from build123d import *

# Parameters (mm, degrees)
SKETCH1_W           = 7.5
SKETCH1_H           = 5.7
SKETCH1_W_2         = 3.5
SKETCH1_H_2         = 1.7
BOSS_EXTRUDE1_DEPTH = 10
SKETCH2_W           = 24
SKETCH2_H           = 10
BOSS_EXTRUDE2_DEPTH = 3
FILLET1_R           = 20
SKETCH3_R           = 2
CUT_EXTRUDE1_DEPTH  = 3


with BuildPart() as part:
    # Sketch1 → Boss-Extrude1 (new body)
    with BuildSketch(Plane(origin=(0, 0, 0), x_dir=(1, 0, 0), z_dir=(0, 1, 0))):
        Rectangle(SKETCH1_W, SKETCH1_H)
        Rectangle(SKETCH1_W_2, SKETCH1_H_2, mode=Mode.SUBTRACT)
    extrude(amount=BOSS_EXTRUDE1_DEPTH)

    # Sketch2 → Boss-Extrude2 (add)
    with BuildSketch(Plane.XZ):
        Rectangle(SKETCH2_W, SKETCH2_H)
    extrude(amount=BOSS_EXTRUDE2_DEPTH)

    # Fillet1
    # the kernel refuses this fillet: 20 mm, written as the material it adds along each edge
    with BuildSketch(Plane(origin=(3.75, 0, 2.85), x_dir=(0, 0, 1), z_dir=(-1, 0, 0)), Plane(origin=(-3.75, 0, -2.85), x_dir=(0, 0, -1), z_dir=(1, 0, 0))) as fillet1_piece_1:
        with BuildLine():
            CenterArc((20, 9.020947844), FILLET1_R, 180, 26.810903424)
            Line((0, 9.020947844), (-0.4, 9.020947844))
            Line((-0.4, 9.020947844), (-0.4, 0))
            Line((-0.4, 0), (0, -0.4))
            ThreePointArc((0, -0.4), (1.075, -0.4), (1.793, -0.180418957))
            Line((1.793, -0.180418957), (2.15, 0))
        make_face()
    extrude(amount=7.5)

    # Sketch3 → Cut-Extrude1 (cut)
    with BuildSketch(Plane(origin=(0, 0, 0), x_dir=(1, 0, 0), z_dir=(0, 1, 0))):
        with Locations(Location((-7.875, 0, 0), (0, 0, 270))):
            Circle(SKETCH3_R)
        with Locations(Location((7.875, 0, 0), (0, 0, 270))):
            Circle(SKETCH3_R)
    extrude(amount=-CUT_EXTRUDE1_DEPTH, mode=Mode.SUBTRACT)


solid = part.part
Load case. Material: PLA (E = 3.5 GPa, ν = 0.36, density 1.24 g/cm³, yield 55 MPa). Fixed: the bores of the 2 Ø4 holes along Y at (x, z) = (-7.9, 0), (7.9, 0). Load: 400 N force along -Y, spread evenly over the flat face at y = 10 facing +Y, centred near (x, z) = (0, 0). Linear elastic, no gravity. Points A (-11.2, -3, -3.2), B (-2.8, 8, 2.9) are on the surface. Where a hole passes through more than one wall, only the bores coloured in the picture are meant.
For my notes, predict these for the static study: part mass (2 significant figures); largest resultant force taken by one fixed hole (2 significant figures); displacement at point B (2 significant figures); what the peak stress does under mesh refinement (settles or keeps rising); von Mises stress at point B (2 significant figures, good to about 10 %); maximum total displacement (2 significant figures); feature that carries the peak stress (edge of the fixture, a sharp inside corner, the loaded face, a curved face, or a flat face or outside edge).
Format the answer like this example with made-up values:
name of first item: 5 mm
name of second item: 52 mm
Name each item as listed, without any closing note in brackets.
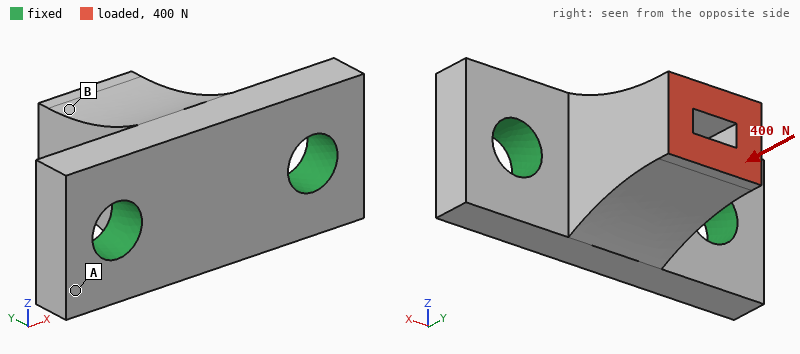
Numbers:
part mass: 1.4 g
largest resultant force taken by one fixed hole: 210 N
displacement at point B: 62 µm
what the peak stress does under mesh refinement: keeps rising
von Mises stress at point B: 12 MPa
maximum total displacement: 69 µm
feature that carries the peak stress: edge of the fixture
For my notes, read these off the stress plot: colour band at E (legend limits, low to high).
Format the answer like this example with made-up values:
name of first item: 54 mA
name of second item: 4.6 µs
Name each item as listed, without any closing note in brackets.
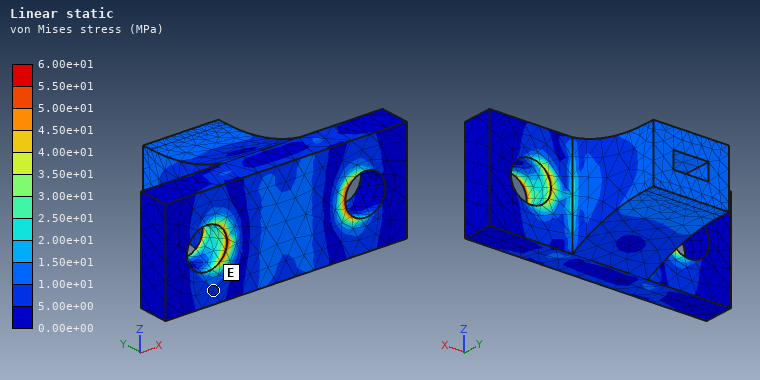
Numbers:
colour band at E: 5.00e+00 to 1.00e+01 MPa
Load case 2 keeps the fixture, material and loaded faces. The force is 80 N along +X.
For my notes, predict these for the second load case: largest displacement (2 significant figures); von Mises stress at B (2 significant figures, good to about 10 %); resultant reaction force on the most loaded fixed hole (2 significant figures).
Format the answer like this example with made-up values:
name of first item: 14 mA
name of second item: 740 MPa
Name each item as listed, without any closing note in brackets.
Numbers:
largest displacement: 96 µm
von Mises stress at B: 3.5 MPa
resultant reaction force on the most loaded fixed hole: 94 N
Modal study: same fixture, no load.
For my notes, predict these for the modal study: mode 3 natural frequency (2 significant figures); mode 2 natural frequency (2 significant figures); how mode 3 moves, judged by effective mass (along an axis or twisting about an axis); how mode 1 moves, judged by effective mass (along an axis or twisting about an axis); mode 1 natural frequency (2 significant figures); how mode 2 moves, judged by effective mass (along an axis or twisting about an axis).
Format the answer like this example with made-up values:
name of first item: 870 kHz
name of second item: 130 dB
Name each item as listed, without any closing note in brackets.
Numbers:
mode 3 natural frequency: 16 kHz
mode 2 natural frequency: 12 kHz
how mode 3 moves, judged by effective mass: along Y
how mode 1 moves, judged by effective mass: along Z
mode 1 natural frequency: 7100 Hz
how mode 2 moves, judged by effective mass: along X
